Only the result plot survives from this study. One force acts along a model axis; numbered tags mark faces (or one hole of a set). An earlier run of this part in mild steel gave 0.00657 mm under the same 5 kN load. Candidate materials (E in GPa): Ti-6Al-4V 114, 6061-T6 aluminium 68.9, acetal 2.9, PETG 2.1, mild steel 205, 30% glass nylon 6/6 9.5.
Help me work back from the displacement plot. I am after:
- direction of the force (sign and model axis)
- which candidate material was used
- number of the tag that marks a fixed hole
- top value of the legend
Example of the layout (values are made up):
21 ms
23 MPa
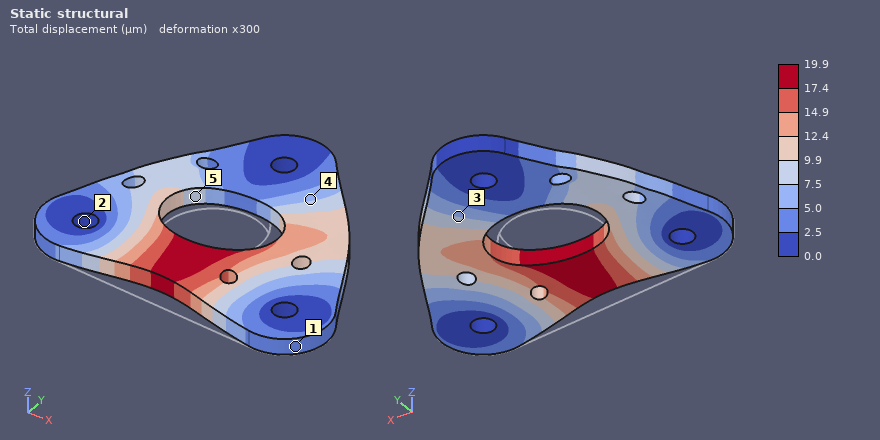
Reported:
+Y
6061-T6 aluminium
2
19.9 µm
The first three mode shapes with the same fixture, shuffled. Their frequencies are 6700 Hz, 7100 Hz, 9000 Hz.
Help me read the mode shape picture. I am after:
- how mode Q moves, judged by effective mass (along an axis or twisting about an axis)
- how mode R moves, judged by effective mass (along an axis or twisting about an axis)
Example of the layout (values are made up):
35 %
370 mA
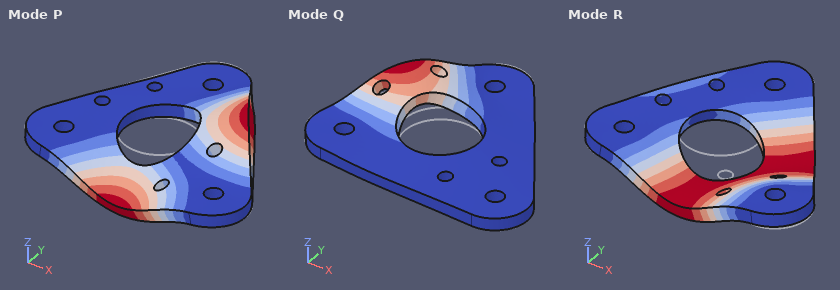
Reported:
along Z
along Z
